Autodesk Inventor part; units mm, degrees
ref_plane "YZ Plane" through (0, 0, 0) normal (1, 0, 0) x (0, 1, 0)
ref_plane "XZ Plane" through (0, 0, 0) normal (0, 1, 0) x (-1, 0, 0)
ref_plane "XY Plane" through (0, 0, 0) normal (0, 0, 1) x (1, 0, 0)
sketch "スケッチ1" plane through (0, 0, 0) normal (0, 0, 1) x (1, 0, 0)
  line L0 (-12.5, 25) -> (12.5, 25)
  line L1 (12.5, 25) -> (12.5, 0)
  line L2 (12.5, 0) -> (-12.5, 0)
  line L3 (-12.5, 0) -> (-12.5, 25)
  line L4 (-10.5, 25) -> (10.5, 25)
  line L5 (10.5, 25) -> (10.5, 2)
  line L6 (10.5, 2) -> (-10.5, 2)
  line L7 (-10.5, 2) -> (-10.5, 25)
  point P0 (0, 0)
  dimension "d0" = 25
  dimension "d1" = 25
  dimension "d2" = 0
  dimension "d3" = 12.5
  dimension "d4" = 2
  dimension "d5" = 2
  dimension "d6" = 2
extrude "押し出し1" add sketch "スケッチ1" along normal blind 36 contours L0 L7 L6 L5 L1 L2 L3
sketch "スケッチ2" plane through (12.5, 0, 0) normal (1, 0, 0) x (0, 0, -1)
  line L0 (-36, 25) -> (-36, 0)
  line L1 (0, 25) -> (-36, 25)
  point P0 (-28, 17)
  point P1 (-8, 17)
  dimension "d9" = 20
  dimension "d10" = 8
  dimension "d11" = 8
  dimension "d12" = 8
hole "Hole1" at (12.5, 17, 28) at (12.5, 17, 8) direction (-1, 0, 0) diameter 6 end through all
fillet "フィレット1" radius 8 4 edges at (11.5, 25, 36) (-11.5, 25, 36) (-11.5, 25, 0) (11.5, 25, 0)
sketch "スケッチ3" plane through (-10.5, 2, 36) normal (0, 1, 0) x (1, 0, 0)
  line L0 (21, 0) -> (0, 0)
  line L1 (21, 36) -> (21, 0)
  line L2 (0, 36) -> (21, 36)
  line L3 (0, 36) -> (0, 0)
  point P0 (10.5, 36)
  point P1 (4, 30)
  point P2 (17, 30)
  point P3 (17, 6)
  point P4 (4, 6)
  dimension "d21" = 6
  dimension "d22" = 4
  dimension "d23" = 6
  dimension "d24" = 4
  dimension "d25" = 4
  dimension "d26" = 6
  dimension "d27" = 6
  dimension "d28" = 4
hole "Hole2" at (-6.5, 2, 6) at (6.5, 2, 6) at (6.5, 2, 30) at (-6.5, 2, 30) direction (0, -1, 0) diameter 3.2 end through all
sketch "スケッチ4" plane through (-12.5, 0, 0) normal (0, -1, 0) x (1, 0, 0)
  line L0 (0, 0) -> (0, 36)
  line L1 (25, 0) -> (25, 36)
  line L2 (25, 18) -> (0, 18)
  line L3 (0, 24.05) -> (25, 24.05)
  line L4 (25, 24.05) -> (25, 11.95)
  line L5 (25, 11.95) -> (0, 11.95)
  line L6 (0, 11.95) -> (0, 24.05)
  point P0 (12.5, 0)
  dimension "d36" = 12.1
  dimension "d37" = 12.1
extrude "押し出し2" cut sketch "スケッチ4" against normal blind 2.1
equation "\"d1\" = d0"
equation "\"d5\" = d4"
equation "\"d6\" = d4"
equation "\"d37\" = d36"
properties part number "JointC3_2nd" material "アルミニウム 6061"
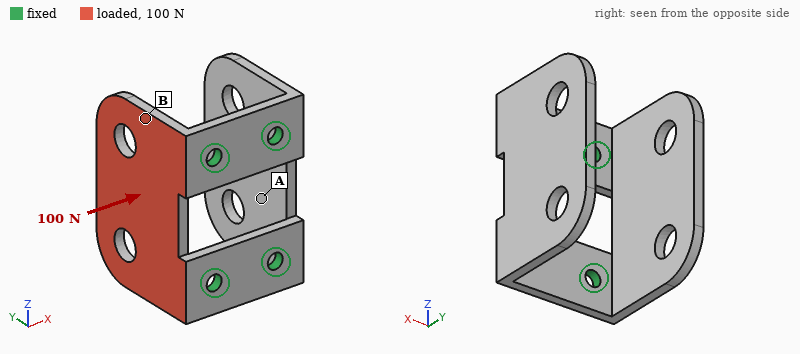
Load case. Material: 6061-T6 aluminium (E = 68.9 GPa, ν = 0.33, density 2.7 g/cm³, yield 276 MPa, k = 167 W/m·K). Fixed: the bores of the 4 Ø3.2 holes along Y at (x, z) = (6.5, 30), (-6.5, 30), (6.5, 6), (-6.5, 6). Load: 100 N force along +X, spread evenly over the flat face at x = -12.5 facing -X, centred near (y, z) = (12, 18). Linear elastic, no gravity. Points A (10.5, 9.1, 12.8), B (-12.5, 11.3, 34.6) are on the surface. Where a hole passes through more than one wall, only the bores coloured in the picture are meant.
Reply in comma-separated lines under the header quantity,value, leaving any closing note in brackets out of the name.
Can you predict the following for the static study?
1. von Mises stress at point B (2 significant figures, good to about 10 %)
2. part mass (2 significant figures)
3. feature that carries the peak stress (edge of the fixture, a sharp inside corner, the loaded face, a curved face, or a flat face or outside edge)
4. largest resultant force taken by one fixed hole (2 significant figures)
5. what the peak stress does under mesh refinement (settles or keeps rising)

quantity,value
von Mises stress at point B,19 MPa
part mass,11 g
feature that carries the peak stress,a sharp inside corner
largest resultant force taken by one fixed hole,47 N
what the peak stress does under mesh refinement,keeps rising
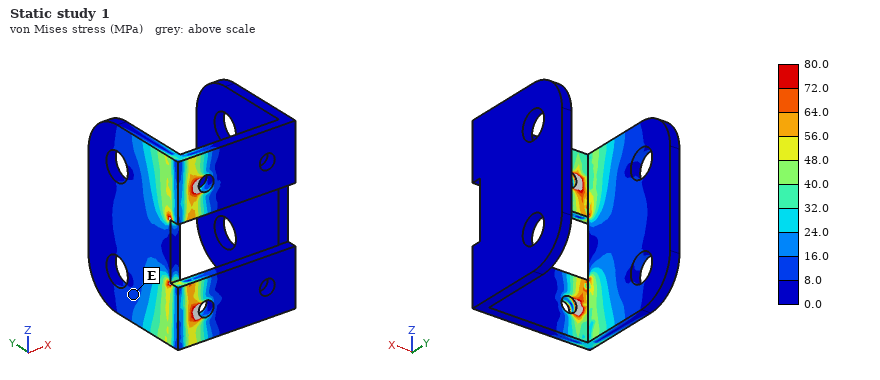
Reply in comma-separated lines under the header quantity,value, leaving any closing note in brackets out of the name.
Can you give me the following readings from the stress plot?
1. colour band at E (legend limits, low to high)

quantity,value
colour band at E,8.0 to 16.0 MPa
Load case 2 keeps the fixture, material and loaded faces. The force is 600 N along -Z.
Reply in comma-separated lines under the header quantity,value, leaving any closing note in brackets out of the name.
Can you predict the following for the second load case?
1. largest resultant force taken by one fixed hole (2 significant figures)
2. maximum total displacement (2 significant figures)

quantity,value
largest resultant force taken by one fixed hole,440 N
maximum total displacement,34 µm
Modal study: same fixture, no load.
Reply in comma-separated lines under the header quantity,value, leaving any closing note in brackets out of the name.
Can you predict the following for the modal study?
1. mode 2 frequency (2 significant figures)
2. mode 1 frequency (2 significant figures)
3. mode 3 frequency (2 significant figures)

quantity,value
mode 2 frequency,2100 Hz
mode 1 frequency,2100 Hz
mode 3 frequency,5000 Hz
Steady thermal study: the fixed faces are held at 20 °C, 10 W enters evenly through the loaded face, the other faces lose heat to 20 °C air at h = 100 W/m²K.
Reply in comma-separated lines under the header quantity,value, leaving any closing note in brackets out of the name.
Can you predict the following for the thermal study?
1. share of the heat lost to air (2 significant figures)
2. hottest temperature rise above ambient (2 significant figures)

quantity,value
share of the heat lost to air,13 %
hottest temperature rise above ambient,15 K
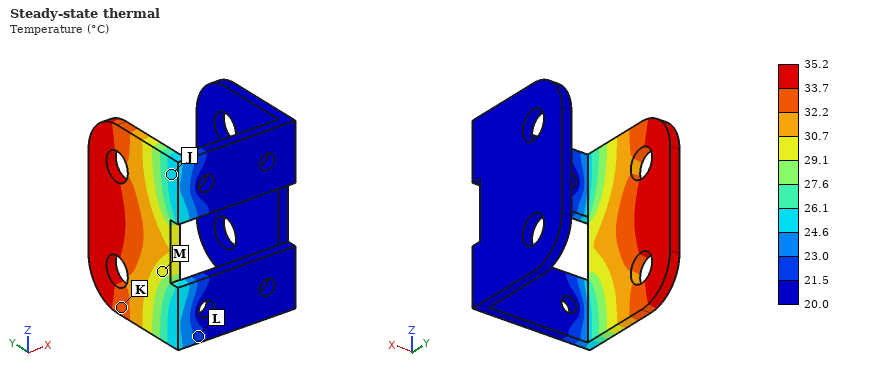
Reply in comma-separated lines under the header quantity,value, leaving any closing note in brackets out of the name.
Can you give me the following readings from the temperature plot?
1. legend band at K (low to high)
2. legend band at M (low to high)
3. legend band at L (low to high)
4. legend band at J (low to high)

quantity,value
legend band at K,32.2 to 33.7 °C
legend band at M,29.1 to 30.7 °C
legend band at L,21.5 to 23.0 °C
legend band at J,24.6 to 26.1 °C
